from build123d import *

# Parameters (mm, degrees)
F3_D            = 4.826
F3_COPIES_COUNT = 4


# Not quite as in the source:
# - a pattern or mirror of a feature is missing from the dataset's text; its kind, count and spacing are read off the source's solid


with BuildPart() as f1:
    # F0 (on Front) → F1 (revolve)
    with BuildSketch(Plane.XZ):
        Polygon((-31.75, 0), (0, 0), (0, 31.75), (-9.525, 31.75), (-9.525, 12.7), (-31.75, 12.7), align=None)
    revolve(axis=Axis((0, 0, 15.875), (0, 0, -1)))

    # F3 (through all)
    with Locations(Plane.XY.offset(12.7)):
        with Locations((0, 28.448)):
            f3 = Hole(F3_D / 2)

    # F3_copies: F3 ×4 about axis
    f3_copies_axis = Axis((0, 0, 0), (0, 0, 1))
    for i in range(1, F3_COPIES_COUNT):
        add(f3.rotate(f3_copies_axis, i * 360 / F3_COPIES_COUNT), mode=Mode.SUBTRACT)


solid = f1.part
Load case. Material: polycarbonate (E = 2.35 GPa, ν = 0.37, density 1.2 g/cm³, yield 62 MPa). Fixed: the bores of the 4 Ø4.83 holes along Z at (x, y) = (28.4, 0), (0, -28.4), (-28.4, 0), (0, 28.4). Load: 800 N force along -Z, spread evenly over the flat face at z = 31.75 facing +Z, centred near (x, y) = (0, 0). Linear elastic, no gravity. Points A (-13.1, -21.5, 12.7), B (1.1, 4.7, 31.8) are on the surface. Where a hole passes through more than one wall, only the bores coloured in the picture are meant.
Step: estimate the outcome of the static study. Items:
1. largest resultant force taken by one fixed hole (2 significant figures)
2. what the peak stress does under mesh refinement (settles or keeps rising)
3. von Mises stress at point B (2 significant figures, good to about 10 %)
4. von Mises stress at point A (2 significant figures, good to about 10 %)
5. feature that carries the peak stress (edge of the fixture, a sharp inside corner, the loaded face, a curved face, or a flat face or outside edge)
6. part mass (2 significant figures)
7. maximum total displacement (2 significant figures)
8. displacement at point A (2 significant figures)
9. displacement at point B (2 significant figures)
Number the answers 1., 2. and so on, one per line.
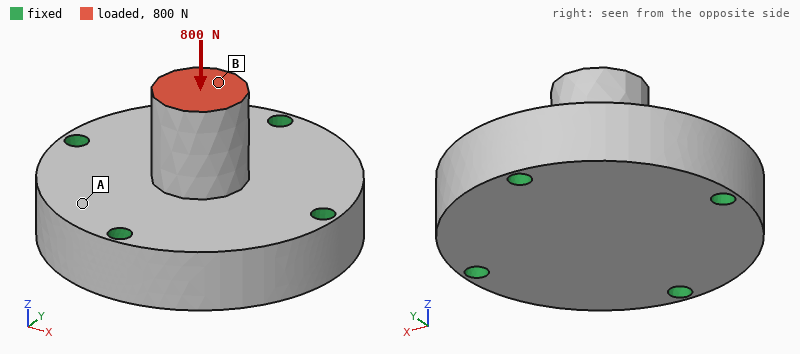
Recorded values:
1. 200 N
2. keeps rising
3. 2.8 MPa
4. 0.92 MPa
5. edge of the fixture
6. 54 g
7. 66 µm
8. 13 µm
9. 65 µm
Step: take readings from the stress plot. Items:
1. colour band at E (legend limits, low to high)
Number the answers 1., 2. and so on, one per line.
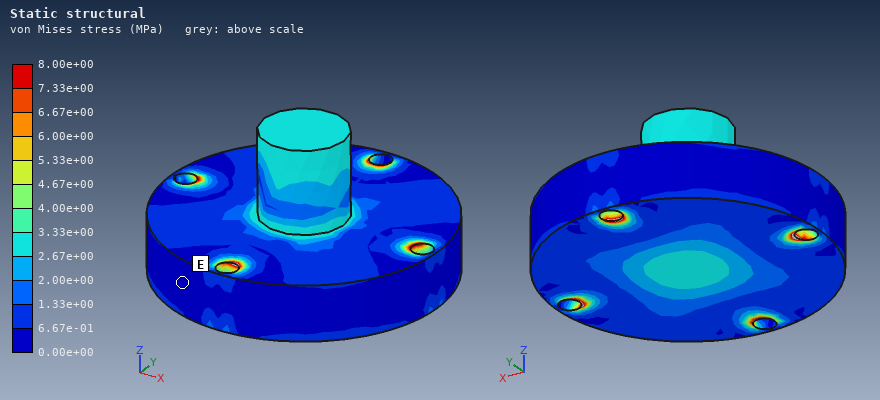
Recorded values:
1. 0.00e+00 to 6.67e-01 MPa
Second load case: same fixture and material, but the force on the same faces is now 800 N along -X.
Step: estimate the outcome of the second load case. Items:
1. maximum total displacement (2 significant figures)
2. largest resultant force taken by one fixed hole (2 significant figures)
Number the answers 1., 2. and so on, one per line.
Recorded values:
1. 0.38 mm
2. 470 N
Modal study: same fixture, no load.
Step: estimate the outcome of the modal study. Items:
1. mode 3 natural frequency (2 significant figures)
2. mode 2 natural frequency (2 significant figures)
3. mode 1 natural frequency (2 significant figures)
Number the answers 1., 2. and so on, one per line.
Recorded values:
1. 4700 Hz
2. 4600 Hz
3. 4600 Hz
